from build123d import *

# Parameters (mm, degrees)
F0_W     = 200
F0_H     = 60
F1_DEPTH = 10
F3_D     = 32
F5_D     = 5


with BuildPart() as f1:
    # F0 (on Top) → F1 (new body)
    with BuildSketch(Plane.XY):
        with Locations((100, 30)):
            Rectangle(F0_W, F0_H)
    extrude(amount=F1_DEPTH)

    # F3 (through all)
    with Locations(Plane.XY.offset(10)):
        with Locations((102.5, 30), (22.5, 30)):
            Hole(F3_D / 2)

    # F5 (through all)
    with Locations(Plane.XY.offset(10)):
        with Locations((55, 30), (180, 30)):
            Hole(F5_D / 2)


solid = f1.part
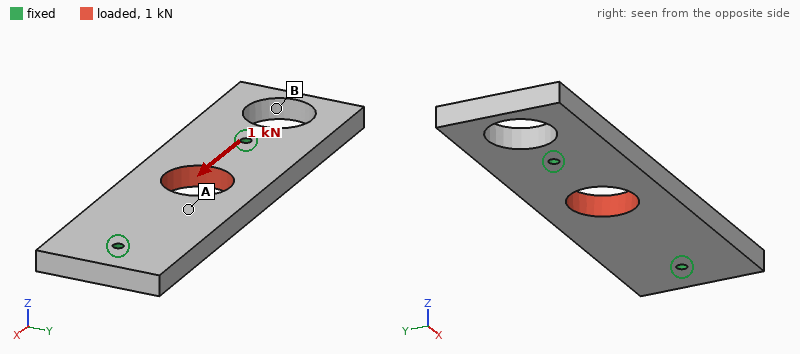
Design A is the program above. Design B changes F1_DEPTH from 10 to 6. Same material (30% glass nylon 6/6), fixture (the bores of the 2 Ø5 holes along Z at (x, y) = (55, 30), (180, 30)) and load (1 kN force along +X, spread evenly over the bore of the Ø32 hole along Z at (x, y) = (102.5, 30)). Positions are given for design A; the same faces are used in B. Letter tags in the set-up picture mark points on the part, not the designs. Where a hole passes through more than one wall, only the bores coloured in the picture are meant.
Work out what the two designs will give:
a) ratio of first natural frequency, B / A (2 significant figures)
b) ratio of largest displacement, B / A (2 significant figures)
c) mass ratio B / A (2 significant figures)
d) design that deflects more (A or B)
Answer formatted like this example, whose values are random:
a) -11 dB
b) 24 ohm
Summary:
a) 0.65
b) 1.7
c) 0.60
d) B
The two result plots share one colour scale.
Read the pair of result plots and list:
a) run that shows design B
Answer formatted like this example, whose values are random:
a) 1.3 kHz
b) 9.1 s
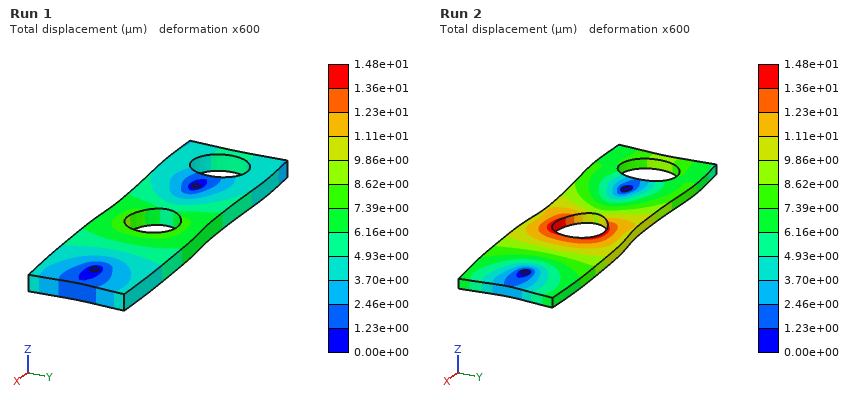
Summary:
a) Run 2
